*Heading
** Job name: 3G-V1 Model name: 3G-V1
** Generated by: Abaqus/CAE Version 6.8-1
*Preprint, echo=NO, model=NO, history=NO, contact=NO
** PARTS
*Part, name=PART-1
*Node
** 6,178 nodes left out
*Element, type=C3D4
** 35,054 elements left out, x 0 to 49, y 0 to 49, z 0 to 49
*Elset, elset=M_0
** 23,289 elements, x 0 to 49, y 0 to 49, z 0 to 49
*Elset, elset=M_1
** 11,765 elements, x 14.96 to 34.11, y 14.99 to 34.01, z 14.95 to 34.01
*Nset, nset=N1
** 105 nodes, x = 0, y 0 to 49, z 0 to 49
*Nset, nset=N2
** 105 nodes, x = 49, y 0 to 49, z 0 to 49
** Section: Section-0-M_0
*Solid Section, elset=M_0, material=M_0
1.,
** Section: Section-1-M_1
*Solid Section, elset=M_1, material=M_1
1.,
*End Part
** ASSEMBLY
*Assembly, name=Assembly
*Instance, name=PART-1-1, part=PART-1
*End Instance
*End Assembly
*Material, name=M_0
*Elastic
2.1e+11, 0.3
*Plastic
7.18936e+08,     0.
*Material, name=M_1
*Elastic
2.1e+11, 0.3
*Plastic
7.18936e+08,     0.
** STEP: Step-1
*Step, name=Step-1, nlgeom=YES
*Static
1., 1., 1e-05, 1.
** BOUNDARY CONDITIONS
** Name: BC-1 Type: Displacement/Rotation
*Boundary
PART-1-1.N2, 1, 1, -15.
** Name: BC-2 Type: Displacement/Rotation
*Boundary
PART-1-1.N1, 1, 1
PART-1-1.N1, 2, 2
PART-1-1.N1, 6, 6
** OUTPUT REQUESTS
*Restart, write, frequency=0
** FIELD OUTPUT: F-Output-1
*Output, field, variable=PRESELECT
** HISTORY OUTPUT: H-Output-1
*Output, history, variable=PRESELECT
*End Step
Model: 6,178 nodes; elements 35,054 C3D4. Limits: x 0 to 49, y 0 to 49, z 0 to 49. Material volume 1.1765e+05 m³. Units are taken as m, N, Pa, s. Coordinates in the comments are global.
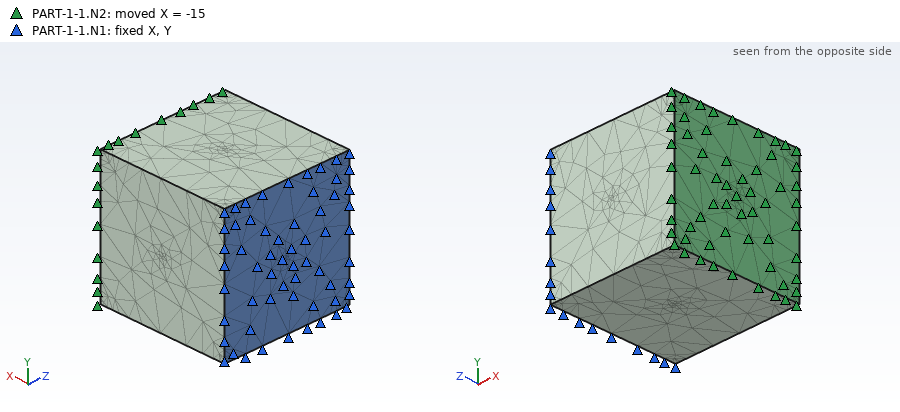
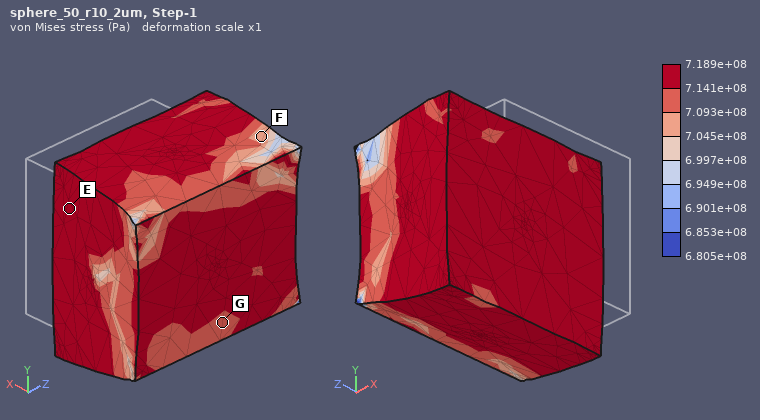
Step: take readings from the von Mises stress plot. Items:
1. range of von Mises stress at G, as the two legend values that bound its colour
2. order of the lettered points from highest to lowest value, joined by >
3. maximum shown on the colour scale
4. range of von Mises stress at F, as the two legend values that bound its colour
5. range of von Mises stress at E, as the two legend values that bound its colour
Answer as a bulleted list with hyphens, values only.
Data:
- 7.093e+08 to 7.141e+08 Pa
- E > G > F
- 7.189e+08 Pa
- 7.045e+08 to 7.093e+08 Pa
- 7.141e+08 to 7.189e+08 Pa
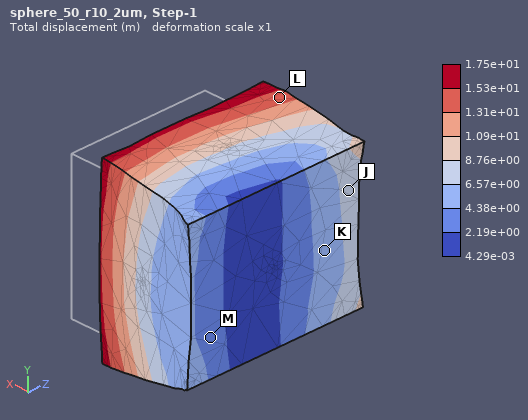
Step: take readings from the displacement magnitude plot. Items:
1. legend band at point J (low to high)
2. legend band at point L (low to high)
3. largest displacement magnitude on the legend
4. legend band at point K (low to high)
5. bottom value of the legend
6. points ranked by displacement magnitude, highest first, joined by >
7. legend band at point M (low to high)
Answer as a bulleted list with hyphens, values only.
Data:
- 6.57e+00 to 8.76e+00 m
- 1.31e+01 to 1.53e+01 m
- 1.75e+01 m
- 4.38e+00 to 6.57e+00 m
- 4.29e-03 m
- L > J > K > M
- 2.19e+00 to 4.38e+00 m
